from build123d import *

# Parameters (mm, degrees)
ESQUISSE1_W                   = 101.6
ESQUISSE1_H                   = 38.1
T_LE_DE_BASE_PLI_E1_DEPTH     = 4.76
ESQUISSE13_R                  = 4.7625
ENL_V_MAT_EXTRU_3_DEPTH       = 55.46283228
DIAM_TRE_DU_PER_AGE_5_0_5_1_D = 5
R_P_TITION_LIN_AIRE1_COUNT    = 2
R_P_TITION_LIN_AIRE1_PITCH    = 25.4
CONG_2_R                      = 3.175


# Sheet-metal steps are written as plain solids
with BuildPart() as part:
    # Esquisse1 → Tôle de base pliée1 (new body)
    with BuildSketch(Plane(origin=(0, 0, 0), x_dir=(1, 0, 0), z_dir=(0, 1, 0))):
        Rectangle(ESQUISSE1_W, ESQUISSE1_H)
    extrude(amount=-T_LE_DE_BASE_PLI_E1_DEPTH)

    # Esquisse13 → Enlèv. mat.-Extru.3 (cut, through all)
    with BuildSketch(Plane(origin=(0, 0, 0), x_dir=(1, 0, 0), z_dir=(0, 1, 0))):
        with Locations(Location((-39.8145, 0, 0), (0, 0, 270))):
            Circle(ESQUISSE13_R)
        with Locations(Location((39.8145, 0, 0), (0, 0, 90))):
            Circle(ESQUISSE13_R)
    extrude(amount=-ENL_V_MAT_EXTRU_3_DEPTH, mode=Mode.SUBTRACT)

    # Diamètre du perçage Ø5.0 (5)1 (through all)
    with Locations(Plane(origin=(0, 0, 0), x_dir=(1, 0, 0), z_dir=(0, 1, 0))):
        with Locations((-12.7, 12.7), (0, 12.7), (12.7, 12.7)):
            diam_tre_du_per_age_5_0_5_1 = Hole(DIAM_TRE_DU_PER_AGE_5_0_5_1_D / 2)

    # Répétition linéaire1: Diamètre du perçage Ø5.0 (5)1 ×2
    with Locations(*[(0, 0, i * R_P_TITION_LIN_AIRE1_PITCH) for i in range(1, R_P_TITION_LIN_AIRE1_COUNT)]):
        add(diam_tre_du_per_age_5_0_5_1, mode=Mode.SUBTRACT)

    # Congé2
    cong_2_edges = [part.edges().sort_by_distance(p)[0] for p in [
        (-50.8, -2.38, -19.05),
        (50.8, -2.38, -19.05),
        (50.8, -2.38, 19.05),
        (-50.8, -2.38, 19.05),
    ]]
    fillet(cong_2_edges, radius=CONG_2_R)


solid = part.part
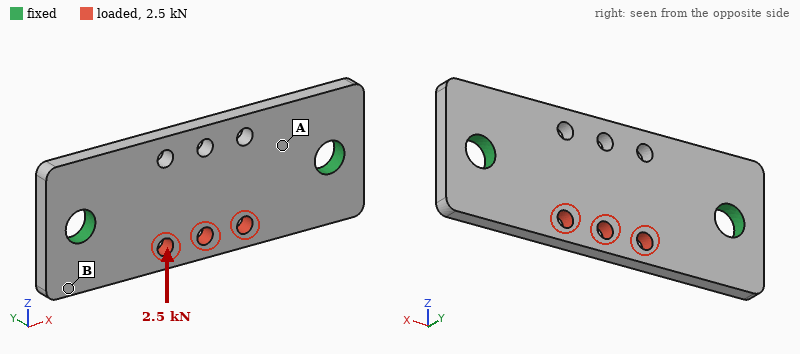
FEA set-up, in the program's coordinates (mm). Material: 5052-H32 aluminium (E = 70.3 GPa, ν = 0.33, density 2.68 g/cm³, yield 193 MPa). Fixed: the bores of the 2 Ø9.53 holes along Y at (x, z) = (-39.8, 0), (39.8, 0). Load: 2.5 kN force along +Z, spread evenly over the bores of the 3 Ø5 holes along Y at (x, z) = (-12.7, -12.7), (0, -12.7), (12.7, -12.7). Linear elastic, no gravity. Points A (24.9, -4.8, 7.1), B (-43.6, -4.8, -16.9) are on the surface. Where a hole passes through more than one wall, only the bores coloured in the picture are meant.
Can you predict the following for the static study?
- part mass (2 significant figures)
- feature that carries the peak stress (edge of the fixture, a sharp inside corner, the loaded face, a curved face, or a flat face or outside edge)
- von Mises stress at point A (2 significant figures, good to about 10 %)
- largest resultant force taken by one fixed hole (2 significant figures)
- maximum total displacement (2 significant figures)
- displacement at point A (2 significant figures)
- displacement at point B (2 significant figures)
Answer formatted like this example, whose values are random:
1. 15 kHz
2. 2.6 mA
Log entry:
1. 46 g
2. edge of the fixture
3. 14 MPa
4. 1.3 kN
5. 21 µm
6. 8.8 µm
7. 5.4 µm
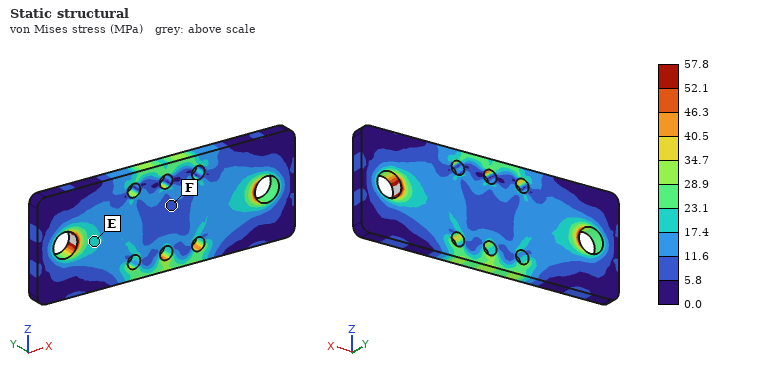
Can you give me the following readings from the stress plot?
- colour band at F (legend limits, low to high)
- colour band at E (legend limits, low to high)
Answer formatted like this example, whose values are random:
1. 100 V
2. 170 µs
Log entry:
1. 5.8 to 11.6 MPa
2. 17.4 to 23.1 MPa
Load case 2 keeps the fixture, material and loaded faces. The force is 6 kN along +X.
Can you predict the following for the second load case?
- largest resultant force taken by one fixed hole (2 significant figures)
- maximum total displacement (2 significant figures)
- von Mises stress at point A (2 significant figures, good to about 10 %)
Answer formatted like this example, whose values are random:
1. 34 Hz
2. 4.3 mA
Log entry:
1. 3.1 kN
2. 18 µm
3. 13 MPa
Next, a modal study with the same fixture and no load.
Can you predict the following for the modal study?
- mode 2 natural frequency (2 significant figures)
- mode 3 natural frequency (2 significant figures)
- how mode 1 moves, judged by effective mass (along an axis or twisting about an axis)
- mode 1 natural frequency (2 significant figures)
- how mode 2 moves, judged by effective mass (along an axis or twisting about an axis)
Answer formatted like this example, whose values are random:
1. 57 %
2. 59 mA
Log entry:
1. 5500 Hz
2. 10 kHz
3. along Y
4. 4200 Hz
5. twisting about X
